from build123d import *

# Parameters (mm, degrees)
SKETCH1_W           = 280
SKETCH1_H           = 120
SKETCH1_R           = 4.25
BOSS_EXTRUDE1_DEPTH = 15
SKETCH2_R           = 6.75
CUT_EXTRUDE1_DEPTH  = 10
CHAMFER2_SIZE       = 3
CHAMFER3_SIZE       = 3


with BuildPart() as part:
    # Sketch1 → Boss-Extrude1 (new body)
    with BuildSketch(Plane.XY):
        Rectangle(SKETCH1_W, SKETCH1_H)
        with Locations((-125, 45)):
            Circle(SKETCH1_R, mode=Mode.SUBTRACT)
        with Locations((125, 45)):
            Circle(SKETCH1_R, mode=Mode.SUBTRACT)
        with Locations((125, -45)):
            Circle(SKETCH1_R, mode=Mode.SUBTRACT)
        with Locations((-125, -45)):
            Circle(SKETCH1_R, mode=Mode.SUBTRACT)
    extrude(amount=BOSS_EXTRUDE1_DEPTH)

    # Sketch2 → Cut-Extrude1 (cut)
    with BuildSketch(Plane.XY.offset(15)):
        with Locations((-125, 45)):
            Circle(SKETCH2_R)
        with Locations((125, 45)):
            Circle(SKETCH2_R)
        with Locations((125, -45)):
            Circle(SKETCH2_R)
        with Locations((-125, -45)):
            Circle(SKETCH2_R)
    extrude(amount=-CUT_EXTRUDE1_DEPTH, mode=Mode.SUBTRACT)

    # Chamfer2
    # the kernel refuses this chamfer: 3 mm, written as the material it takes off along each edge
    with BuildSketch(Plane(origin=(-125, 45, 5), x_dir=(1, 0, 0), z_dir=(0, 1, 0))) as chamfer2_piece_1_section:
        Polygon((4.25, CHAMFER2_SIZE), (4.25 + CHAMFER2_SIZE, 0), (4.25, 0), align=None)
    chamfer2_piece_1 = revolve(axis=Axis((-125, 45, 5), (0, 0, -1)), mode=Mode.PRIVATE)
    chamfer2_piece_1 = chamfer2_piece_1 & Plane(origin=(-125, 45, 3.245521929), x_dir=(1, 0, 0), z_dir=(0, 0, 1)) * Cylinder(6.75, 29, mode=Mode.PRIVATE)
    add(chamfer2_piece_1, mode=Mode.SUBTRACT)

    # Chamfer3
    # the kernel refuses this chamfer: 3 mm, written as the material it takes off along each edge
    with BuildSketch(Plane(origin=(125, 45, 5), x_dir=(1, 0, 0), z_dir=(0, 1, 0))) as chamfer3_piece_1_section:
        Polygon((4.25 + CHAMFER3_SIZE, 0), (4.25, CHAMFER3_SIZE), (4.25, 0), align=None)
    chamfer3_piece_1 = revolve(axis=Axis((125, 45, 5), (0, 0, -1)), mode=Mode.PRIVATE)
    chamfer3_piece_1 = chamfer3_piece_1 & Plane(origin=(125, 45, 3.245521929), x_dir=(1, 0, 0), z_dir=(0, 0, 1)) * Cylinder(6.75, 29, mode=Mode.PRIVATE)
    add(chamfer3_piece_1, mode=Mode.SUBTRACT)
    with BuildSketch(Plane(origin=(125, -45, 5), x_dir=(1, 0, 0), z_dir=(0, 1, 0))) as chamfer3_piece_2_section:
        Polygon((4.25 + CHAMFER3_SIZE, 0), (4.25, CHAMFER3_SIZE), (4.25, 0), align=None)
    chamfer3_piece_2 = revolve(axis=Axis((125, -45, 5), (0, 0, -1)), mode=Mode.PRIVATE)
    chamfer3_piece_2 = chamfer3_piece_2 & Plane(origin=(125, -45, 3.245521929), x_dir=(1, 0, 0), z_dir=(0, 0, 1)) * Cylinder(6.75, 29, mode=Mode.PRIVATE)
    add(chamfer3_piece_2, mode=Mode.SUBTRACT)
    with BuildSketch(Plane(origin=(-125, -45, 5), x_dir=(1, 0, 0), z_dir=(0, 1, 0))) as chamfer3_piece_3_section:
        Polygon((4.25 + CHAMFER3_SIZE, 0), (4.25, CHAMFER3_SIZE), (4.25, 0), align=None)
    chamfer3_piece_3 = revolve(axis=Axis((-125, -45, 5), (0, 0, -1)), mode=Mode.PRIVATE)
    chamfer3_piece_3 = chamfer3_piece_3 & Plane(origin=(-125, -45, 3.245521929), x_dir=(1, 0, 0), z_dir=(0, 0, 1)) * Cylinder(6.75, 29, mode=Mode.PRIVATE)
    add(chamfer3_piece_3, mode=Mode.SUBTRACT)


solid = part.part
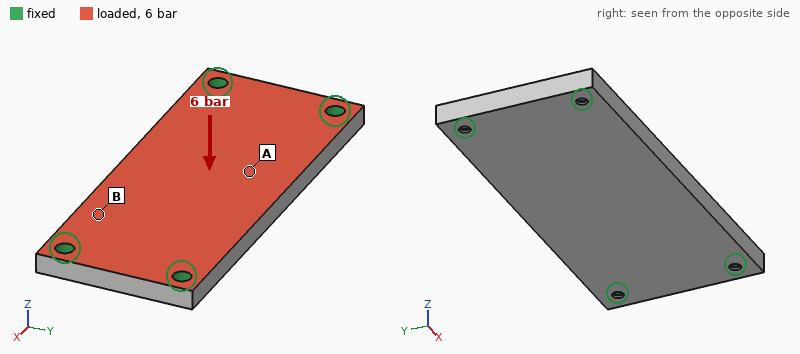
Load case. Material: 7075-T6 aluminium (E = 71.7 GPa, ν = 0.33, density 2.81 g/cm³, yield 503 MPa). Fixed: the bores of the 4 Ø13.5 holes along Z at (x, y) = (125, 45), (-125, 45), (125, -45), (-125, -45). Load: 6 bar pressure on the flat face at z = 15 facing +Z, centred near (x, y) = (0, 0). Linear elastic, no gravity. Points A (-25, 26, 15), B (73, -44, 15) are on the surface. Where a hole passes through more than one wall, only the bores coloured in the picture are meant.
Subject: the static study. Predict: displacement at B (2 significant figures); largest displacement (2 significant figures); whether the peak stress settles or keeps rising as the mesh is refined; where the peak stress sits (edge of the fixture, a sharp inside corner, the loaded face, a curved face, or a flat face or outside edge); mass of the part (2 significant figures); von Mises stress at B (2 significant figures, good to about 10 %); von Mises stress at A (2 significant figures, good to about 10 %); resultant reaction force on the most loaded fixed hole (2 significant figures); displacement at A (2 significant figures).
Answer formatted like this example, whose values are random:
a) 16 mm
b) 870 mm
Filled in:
a) 0.18 mm
b) 0.39 mm
c) keeps rising
d) edge of the fixture
e) 1.4 kg
f) 13 MPa
g) 37 MPa
h) 5.1 kN
i) 0.34 mm
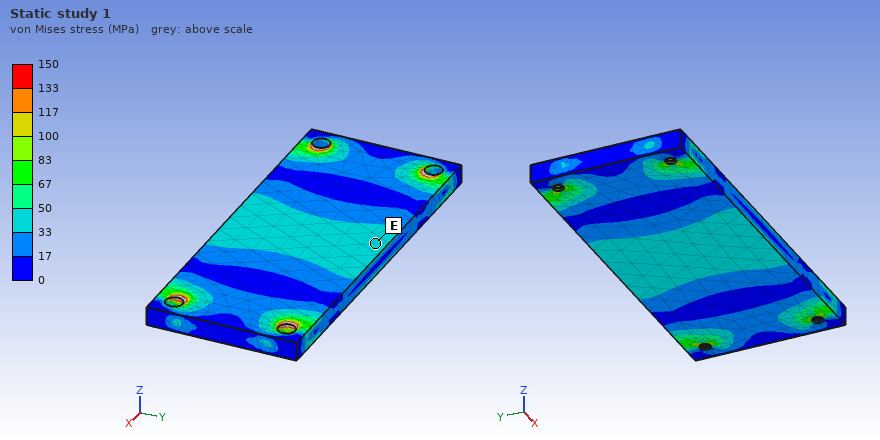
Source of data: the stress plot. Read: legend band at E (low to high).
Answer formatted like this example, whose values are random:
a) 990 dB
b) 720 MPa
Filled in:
a) 33 to 50 MPa
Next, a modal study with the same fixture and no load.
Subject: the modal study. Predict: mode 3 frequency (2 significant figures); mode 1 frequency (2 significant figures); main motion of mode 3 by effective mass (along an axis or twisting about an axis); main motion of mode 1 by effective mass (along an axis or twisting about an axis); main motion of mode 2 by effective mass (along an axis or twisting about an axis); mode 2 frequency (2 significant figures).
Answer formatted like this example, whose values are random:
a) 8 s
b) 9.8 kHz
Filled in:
a) 3100 Hz
b) 1100 Hz
c) twisting about Y
d) along Z
e) twisting about X
f) 2000 Hz
